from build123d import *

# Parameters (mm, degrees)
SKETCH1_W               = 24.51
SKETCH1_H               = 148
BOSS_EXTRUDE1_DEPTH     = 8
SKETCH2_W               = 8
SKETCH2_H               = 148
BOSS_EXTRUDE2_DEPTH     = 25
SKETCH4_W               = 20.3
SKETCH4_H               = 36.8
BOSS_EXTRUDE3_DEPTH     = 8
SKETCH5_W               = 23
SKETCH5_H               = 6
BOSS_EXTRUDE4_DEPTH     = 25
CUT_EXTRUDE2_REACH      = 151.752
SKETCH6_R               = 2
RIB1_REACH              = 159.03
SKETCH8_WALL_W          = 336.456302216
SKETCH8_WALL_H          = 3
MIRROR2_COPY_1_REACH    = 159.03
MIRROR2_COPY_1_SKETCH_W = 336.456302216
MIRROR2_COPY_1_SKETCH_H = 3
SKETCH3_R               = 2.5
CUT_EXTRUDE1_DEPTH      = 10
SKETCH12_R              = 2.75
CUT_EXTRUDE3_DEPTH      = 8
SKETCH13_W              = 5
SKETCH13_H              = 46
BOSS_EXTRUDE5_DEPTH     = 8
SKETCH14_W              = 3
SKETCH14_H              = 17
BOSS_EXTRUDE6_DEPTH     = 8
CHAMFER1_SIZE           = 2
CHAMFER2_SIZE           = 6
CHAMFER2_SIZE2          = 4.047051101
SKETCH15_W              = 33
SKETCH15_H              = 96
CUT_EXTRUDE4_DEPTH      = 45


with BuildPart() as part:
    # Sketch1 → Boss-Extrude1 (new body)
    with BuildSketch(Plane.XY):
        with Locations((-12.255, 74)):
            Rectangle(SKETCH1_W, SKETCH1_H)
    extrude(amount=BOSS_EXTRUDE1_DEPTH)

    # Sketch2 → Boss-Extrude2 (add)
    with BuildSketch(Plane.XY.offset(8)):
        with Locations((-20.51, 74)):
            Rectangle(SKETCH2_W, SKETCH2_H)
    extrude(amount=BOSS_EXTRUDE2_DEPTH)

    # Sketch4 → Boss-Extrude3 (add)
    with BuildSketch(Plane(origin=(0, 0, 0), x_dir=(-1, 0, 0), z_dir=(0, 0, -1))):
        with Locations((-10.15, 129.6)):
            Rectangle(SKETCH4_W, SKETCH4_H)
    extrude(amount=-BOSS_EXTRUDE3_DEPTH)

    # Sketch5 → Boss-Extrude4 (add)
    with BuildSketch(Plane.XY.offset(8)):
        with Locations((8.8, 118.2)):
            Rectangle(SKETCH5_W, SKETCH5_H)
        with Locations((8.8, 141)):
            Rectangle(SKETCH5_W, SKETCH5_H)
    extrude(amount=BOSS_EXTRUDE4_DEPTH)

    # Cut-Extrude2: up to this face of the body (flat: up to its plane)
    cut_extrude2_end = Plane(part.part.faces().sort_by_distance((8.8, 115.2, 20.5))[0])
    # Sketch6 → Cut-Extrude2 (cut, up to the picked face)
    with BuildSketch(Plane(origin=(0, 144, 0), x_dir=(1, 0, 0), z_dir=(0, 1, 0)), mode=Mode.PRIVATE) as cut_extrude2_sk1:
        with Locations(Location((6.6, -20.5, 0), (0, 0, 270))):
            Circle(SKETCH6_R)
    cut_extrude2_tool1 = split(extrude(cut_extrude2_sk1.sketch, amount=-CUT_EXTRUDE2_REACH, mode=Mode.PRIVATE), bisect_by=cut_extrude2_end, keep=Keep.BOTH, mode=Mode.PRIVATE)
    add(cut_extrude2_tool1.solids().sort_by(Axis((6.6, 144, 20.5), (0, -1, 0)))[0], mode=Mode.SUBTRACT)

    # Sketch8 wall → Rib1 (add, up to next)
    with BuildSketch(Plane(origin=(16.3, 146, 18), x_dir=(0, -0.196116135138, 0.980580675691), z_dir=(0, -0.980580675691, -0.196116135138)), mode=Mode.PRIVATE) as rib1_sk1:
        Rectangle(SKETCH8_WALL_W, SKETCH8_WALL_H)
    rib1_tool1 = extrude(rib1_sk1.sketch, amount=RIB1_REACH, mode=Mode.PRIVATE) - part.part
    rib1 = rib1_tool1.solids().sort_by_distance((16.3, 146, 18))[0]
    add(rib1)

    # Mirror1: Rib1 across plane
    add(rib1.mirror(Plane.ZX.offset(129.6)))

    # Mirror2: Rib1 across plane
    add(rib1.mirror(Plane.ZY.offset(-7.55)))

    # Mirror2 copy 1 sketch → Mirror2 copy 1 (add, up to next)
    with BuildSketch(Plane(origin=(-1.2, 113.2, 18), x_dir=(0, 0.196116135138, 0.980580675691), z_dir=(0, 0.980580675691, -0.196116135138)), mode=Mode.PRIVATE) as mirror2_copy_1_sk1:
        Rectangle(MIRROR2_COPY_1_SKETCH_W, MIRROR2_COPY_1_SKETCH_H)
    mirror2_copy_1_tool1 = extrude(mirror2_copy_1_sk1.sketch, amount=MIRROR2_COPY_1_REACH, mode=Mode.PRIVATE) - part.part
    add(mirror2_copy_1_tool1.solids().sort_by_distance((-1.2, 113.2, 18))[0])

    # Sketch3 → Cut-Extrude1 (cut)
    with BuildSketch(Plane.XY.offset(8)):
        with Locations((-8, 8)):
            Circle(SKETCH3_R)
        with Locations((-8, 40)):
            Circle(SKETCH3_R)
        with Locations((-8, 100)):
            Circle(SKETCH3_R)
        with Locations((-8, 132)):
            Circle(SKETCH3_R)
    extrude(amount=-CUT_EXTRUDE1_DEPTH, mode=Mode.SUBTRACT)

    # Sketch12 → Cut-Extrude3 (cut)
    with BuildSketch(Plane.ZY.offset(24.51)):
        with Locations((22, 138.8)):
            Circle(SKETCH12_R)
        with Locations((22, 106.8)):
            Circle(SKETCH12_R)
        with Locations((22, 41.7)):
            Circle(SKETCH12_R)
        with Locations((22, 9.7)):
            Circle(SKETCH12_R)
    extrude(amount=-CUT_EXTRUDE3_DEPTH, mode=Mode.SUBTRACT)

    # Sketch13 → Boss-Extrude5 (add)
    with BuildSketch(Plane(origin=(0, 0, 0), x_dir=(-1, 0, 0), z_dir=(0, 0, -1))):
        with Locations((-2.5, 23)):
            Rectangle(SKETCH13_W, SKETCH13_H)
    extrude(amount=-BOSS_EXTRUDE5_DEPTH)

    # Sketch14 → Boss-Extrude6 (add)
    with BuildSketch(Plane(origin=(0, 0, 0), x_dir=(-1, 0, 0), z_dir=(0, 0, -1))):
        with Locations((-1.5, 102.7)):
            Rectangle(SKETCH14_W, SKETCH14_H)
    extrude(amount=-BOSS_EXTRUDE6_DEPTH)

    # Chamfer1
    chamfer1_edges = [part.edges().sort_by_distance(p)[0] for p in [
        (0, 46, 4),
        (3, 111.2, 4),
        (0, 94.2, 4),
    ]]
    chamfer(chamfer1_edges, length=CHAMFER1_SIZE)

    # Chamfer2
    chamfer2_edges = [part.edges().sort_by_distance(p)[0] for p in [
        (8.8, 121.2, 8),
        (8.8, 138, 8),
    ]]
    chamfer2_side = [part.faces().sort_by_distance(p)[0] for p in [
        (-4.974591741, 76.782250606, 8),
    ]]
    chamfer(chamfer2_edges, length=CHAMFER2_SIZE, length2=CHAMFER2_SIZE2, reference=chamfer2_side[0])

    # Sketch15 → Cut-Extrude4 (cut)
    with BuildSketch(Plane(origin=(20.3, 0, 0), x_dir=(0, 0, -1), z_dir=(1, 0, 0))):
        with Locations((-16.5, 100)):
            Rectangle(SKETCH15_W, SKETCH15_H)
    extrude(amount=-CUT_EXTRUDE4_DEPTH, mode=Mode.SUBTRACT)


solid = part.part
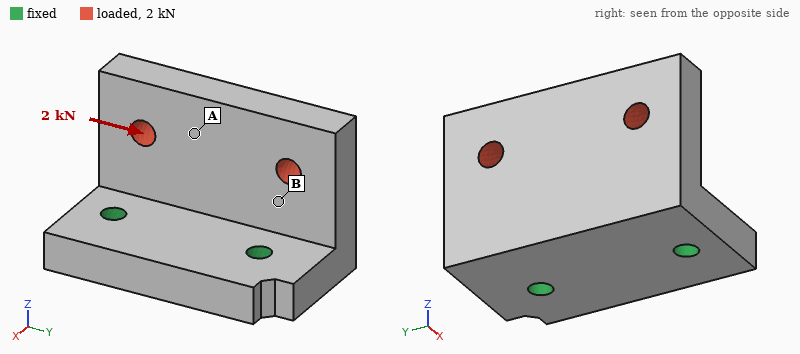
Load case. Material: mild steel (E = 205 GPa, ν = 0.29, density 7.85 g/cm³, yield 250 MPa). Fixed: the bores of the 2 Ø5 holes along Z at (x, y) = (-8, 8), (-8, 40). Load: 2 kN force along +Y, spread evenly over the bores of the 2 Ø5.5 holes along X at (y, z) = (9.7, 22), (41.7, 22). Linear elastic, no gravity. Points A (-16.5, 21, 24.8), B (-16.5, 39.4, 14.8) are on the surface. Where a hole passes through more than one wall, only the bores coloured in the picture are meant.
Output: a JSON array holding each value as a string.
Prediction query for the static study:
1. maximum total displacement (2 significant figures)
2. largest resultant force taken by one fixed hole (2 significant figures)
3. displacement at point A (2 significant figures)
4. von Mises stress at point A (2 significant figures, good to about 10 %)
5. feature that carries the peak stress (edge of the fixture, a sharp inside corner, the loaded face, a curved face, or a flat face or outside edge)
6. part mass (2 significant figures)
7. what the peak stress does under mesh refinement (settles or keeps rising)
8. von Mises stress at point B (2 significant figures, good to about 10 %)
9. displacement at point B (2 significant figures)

["9.2 µm", "1.6 kN", "5.7 µm", "8.5 MPa", "edge of the fixture", "170 g", "keeps rising", "19 MPa", "4.0 µm"]
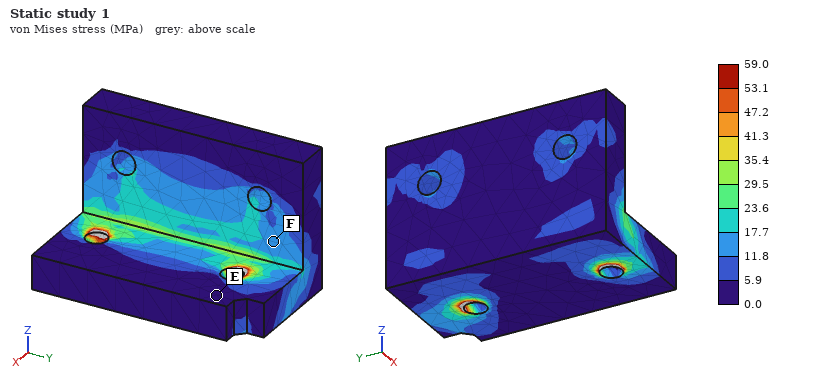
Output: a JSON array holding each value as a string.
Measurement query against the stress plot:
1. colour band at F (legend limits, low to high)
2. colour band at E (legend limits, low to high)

["11.8 to 17.7 MPa", "0.0 to 5.9 MPa"]
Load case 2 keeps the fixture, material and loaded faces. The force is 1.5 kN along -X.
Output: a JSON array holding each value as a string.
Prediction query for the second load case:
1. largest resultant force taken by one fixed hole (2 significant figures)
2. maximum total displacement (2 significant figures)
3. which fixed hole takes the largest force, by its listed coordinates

["830 N", "33 µm", "(-8, 40)"]
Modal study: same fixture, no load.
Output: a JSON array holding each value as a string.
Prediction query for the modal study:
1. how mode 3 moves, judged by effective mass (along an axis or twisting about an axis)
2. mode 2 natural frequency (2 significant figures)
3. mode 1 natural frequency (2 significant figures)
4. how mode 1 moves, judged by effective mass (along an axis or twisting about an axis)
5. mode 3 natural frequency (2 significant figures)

["along Y", "8500 Hz", "4600 Hz", "along X", "12 kHz"]
